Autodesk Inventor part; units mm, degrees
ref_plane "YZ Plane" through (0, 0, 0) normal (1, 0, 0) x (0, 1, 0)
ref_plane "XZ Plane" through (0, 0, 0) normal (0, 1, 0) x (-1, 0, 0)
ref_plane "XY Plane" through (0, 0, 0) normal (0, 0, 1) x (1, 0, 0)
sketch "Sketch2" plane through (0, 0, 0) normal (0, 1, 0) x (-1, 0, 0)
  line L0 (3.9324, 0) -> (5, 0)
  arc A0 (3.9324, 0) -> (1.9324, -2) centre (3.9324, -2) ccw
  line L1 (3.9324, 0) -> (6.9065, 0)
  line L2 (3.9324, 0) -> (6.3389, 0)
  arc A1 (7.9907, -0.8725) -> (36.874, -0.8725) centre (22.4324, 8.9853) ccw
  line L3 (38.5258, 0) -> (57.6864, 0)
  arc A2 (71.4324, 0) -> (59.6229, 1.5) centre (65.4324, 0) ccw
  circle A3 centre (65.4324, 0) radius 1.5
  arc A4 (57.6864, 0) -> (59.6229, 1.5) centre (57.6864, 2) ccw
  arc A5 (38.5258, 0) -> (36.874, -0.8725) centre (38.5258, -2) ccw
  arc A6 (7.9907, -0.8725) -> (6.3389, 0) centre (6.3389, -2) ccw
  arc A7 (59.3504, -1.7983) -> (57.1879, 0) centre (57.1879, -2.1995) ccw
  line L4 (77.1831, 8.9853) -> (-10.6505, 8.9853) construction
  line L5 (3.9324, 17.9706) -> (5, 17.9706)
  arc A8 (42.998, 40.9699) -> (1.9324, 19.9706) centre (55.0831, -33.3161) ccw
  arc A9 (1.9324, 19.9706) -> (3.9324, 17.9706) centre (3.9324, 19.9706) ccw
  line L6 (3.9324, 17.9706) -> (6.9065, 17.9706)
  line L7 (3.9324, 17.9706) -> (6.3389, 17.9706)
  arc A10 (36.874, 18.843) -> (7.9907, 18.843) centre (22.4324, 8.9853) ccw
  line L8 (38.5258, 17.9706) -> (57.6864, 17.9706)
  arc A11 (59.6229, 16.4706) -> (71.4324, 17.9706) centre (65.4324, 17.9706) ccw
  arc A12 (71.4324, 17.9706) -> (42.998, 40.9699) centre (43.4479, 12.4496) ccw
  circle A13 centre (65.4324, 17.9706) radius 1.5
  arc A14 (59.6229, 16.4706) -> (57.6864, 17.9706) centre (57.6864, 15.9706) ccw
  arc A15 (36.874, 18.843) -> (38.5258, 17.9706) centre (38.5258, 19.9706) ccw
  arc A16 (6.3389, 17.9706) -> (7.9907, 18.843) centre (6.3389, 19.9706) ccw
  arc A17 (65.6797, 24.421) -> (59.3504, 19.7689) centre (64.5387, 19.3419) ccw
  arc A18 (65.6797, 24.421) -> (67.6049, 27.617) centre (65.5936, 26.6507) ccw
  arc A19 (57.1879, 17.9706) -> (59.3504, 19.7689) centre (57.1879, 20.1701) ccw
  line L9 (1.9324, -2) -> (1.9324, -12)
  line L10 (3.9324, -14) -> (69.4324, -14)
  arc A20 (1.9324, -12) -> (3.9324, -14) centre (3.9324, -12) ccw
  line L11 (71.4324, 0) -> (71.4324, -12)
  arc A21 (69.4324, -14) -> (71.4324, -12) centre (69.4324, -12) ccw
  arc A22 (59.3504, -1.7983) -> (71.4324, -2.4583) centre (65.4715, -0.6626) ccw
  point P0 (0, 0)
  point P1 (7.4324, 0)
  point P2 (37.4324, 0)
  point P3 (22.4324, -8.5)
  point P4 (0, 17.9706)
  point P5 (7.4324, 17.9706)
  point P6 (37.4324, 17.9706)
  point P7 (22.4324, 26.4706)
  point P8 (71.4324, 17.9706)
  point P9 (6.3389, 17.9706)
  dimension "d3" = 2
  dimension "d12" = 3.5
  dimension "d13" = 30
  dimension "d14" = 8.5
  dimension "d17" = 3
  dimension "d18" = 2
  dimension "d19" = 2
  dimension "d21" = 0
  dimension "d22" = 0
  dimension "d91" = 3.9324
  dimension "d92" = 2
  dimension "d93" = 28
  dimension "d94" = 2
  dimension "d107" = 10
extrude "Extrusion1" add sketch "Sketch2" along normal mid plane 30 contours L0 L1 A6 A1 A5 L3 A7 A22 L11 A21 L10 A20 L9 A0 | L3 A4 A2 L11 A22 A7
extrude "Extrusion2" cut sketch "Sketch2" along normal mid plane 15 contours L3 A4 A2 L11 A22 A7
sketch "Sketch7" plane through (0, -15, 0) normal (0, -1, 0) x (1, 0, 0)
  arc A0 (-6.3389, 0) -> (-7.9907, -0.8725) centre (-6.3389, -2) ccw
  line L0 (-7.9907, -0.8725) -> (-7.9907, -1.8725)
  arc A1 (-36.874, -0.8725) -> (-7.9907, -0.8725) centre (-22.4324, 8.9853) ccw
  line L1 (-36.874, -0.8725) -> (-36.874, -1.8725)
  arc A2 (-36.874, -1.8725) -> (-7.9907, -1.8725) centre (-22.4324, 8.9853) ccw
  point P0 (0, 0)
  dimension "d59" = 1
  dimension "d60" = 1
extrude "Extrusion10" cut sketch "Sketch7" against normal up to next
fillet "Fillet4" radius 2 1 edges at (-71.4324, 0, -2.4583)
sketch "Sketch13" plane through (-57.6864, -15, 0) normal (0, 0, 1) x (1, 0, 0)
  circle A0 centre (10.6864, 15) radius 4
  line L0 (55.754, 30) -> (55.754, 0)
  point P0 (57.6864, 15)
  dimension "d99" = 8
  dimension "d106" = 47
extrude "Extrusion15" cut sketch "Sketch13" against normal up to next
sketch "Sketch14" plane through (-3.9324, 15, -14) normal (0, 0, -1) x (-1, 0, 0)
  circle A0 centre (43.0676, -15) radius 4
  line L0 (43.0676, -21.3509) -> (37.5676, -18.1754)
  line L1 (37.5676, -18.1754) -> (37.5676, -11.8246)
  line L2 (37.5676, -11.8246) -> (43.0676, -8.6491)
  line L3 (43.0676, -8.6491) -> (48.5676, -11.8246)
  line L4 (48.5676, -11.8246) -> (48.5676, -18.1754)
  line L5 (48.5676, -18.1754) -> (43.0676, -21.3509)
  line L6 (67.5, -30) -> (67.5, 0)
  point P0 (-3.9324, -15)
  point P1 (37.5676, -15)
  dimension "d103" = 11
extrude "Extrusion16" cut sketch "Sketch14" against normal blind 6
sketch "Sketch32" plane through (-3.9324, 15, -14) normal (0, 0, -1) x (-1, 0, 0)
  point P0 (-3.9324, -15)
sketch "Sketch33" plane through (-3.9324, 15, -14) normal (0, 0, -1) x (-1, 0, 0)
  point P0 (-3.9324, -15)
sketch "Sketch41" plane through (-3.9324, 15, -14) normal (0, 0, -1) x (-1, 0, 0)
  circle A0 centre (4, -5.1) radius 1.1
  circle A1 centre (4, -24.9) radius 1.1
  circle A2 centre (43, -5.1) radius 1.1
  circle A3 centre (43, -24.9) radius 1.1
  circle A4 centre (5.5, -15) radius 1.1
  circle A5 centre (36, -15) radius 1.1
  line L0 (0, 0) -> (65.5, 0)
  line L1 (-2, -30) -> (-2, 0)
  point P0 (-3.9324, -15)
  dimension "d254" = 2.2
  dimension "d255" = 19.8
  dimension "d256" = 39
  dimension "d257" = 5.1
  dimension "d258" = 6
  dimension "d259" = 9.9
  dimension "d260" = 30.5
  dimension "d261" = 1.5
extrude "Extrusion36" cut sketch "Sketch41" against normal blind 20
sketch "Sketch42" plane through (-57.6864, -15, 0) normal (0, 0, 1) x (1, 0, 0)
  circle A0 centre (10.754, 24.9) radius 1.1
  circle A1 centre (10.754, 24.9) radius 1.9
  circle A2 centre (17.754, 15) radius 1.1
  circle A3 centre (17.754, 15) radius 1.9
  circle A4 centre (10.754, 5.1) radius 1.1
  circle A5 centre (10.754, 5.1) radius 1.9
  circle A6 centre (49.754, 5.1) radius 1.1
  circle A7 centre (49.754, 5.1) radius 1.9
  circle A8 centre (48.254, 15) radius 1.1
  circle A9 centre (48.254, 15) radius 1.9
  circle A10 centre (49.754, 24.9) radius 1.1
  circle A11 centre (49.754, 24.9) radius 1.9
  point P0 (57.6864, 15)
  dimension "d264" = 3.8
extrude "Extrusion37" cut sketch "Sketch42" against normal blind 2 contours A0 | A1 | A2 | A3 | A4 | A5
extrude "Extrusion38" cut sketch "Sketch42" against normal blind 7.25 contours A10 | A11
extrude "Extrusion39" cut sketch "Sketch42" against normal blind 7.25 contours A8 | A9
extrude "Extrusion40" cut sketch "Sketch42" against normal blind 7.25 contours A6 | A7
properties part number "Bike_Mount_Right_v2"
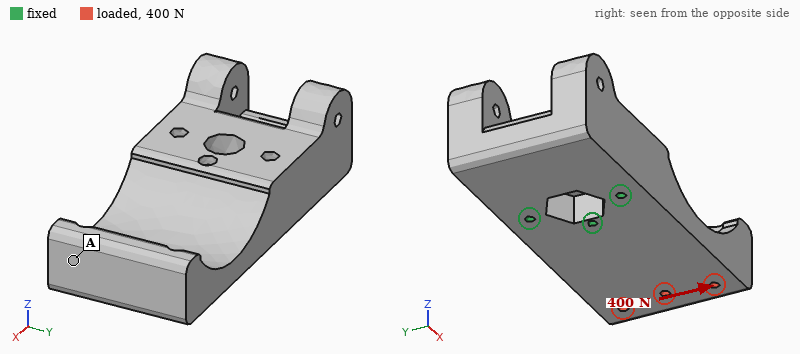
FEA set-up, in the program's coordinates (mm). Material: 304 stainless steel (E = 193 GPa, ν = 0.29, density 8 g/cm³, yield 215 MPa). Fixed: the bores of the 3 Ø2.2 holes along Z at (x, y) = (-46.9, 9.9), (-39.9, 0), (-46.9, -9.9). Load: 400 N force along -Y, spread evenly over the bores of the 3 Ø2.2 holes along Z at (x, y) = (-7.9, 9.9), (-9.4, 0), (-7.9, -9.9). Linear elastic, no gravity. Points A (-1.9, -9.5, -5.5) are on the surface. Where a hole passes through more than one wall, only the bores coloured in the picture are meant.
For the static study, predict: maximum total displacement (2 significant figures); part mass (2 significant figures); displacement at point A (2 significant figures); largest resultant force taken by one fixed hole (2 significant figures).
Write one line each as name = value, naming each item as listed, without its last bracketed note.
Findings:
maximum total displacement = 4.8 µm
part mass = 170 g
displacement at point A = 4.4 µm
largest resultant force taken by one fixed hole = 590 N
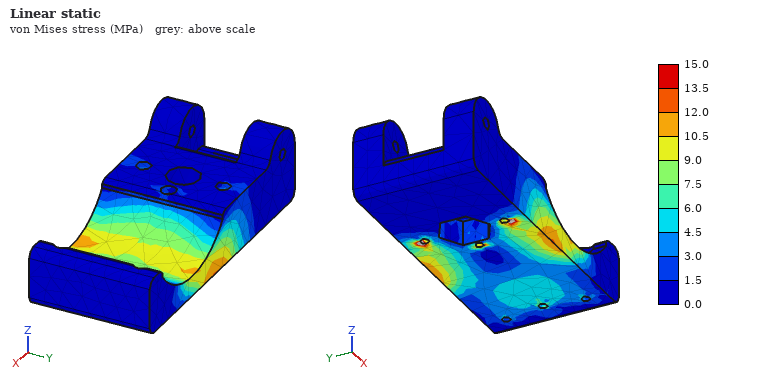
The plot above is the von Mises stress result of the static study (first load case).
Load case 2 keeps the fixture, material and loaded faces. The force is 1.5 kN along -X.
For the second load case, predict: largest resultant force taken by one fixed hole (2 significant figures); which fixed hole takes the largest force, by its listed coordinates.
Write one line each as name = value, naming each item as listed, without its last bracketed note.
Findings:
largest resultant force taken by one fixed hole = 590 N
which fixed hole takes the largest force, by its listed coordinates = (-39.9, 0)
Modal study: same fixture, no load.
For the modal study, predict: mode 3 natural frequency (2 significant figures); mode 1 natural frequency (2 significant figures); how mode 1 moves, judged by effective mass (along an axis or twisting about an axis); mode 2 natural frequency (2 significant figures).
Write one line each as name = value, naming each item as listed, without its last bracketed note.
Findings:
mode 3 natural frequency = 9700 Hz
mode 1 natural frequency = 2900 Hz
how mode 1 moves, judged by effective mass = along Z
mode 2 natural frequency = 6700 Hz
